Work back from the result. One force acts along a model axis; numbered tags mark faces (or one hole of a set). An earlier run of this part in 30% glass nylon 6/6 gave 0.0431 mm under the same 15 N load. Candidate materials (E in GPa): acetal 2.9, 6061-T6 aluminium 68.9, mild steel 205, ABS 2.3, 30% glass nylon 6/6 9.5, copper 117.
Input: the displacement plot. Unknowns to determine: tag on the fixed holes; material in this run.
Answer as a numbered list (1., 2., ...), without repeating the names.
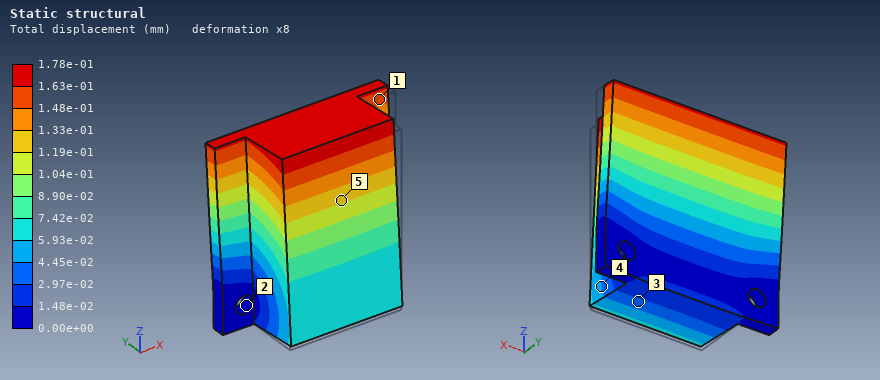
1. 2
2. ABS
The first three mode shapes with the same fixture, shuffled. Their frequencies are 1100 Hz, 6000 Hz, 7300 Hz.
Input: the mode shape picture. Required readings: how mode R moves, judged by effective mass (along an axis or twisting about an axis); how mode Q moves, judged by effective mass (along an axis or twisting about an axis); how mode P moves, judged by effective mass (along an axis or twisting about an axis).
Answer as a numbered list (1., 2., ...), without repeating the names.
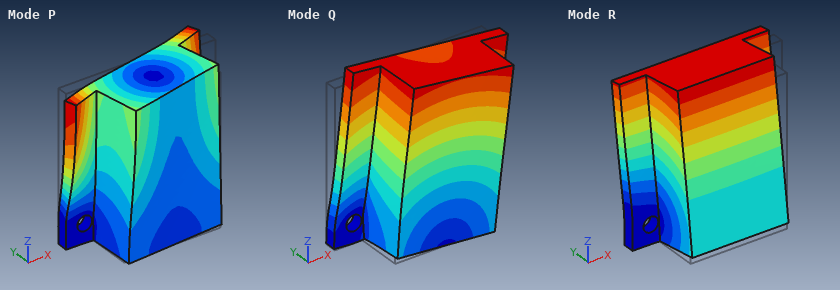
1. along Y
2. along X
3. twisting about Z
